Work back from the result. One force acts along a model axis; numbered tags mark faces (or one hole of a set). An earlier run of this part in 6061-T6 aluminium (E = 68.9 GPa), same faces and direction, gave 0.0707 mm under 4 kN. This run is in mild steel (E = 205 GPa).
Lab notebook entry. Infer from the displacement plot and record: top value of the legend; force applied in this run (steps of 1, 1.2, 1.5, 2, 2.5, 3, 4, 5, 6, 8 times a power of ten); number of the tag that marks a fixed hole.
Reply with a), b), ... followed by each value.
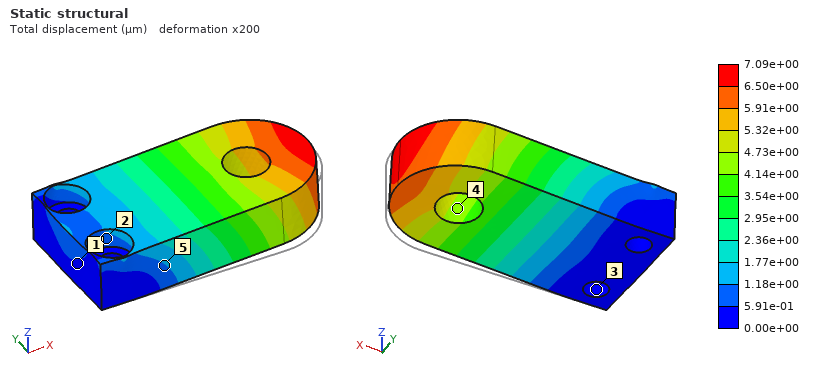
a) 7.09e+00 µm
b) 1.2 kN
c) 3
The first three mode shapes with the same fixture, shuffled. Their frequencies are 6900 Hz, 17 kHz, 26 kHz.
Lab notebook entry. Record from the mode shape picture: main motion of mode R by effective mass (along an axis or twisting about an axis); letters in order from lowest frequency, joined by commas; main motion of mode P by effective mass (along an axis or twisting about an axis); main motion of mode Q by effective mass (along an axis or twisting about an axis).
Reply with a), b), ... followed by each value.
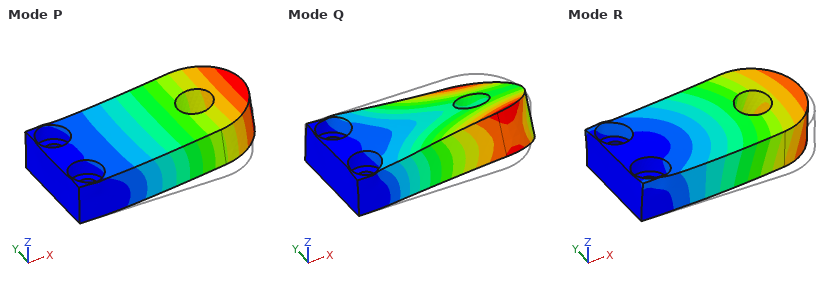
a) along Y
b) P, R, Q
c) along Z
d) twisting about X
